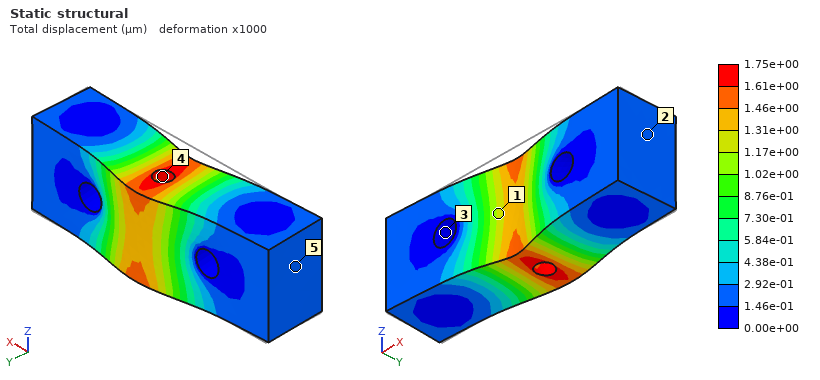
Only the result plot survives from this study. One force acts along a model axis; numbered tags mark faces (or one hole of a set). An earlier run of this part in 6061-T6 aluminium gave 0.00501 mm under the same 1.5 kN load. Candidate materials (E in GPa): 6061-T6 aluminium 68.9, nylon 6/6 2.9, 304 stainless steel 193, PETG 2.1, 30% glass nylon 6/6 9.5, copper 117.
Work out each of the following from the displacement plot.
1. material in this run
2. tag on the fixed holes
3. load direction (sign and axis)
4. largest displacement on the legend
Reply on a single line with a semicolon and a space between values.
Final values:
304 stainless steel; 3; +Y; 1.75e+00 µm
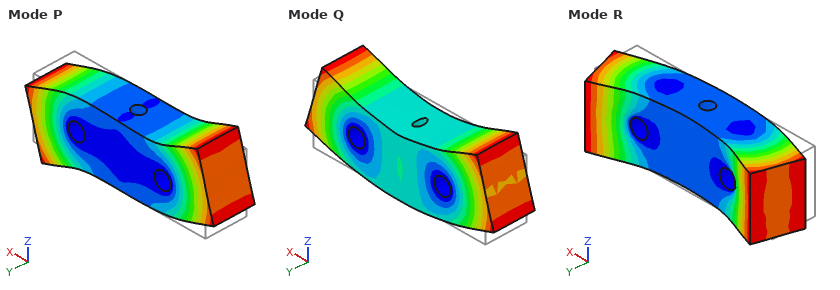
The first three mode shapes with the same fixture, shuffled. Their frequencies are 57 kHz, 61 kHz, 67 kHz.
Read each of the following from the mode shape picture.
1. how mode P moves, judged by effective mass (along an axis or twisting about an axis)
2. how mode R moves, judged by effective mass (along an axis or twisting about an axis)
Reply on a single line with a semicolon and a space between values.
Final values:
twisting about Y; along Y
